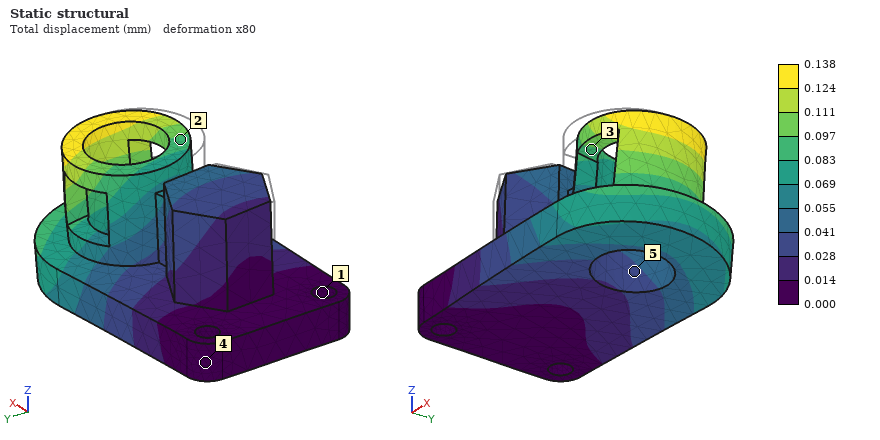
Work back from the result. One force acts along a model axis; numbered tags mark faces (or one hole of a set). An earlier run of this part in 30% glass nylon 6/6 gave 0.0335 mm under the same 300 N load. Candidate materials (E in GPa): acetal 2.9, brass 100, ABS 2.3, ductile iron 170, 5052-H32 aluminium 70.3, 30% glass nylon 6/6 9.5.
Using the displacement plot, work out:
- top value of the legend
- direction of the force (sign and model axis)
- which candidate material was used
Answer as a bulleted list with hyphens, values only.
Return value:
- 0.138 mm
- +Y
- ABS
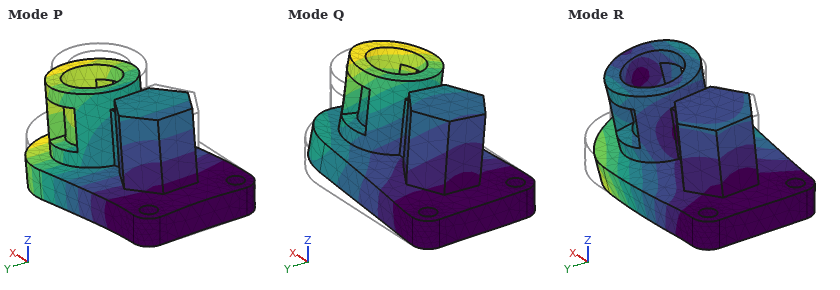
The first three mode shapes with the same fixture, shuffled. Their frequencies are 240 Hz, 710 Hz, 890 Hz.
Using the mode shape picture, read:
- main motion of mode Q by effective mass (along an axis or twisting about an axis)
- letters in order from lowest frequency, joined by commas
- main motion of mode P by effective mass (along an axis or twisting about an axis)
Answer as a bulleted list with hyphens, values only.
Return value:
- along Y
- P, Q, R
- along Z
